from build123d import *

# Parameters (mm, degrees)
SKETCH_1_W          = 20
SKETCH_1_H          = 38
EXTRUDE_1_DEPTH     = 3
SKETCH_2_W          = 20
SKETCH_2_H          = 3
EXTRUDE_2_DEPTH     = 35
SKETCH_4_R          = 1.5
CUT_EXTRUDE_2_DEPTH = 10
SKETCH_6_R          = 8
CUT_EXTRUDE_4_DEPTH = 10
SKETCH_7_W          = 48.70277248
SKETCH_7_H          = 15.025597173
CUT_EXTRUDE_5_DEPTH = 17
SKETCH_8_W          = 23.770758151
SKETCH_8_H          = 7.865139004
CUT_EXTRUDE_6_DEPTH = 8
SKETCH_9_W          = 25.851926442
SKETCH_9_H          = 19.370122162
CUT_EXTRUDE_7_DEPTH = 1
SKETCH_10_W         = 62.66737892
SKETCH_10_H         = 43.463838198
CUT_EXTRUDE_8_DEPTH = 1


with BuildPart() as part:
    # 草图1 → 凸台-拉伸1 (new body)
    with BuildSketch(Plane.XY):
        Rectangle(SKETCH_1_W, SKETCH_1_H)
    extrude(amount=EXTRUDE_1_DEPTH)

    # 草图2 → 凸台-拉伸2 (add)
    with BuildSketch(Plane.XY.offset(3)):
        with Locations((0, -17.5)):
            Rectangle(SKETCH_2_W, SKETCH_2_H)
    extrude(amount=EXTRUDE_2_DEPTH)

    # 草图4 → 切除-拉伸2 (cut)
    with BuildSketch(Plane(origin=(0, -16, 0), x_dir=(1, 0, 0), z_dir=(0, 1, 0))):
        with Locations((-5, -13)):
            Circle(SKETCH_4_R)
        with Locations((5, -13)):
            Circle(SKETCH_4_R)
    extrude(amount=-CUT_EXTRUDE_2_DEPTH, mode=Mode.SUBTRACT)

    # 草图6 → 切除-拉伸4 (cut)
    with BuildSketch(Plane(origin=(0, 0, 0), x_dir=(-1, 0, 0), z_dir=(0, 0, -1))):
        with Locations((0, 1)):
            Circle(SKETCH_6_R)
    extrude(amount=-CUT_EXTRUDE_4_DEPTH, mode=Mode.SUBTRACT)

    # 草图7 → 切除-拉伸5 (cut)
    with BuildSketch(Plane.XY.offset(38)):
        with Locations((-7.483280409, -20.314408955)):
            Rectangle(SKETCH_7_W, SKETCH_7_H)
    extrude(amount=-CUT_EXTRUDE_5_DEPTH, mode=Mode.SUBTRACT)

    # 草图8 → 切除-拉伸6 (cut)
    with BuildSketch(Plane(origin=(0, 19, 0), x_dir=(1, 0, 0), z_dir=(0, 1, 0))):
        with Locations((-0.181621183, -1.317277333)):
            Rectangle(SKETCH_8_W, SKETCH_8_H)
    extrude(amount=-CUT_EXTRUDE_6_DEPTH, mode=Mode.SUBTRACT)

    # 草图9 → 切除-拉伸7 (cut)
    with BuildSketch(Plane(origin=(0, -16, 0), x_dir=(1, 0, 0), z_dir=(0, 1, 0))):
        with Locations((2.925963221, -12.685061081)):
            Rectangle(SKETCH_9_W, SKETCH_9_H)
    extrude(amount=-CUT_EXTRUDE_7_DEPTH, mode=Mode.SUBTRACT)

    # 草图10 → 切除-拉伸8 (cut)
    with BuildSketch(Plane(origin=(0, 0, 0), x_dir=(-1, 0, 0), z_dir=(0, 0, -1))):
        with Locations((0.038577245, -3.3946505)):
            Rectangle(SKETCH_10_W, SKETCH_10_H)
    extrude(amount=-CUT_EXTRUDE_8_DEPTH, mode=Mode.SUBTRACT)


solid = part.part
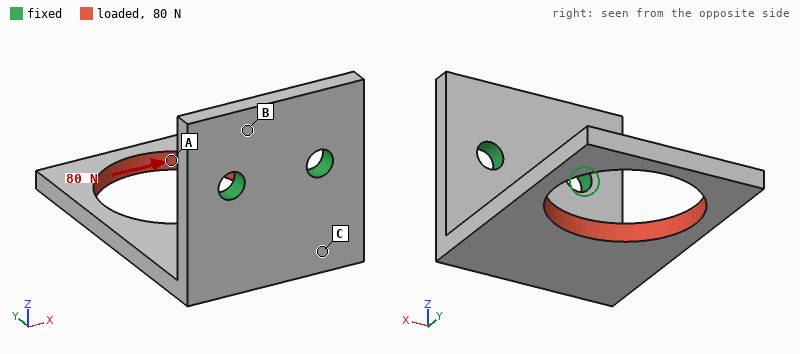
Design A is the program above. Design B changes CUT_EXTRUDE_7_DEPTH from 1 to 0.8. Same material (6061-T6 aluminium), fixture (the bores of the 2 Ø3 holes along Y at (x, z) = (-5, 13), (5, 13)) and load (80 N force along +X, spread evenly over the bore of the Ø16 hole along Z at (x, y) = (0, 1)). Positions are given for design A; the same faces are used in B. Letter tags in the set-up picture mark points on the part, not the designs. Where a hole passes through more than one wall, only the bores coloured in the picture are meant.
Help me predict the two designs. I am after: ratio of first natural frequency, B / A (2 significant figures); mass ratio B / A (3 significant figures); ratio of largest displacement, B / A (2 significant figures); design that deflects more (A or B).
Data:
1.1
1.05
0.82
A
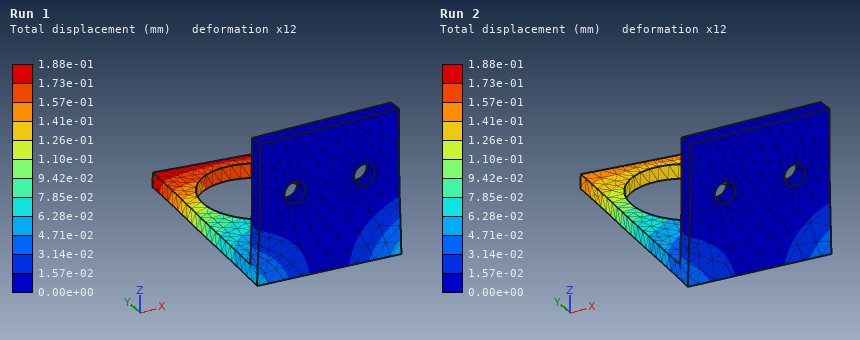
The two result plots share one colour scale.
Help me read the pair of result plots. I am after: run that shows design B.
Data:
Run 2
